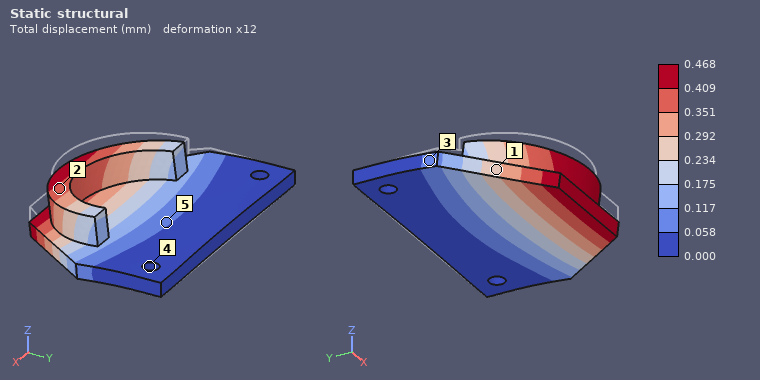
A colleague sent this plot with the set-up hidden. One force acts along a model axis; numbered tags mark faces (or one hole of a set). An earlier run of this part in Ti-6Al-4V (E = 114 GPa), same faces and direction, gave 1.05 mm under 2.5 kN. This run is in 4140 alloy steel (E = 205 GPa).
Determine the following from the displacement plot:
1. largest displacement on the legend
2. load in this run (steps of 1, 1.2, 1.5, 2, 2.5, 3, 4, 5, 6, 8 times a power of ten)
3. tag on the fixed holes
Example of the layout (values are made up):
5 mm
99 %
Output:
0.468 mm
2 kN
4
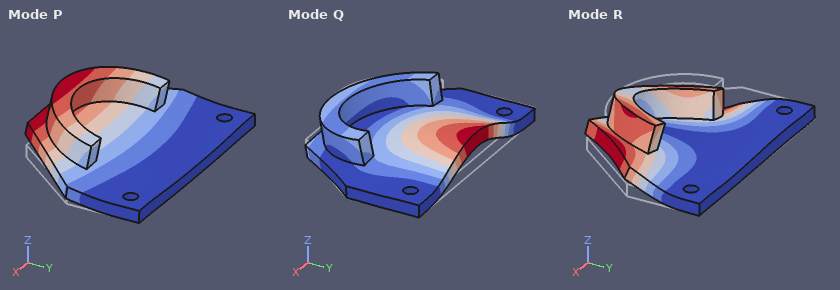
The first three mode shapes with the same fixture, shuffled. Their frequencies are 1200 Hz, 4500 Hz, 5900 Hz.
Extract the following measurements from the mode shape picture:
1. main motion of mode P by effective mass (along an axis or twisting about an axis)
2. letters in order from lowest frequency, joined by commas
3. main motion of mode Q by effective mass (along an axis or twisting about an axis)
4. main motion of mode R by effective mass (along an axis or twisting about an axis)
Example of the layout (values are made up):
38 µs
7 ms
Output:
along Z
P, R, Q
along Z
twisting about Y
